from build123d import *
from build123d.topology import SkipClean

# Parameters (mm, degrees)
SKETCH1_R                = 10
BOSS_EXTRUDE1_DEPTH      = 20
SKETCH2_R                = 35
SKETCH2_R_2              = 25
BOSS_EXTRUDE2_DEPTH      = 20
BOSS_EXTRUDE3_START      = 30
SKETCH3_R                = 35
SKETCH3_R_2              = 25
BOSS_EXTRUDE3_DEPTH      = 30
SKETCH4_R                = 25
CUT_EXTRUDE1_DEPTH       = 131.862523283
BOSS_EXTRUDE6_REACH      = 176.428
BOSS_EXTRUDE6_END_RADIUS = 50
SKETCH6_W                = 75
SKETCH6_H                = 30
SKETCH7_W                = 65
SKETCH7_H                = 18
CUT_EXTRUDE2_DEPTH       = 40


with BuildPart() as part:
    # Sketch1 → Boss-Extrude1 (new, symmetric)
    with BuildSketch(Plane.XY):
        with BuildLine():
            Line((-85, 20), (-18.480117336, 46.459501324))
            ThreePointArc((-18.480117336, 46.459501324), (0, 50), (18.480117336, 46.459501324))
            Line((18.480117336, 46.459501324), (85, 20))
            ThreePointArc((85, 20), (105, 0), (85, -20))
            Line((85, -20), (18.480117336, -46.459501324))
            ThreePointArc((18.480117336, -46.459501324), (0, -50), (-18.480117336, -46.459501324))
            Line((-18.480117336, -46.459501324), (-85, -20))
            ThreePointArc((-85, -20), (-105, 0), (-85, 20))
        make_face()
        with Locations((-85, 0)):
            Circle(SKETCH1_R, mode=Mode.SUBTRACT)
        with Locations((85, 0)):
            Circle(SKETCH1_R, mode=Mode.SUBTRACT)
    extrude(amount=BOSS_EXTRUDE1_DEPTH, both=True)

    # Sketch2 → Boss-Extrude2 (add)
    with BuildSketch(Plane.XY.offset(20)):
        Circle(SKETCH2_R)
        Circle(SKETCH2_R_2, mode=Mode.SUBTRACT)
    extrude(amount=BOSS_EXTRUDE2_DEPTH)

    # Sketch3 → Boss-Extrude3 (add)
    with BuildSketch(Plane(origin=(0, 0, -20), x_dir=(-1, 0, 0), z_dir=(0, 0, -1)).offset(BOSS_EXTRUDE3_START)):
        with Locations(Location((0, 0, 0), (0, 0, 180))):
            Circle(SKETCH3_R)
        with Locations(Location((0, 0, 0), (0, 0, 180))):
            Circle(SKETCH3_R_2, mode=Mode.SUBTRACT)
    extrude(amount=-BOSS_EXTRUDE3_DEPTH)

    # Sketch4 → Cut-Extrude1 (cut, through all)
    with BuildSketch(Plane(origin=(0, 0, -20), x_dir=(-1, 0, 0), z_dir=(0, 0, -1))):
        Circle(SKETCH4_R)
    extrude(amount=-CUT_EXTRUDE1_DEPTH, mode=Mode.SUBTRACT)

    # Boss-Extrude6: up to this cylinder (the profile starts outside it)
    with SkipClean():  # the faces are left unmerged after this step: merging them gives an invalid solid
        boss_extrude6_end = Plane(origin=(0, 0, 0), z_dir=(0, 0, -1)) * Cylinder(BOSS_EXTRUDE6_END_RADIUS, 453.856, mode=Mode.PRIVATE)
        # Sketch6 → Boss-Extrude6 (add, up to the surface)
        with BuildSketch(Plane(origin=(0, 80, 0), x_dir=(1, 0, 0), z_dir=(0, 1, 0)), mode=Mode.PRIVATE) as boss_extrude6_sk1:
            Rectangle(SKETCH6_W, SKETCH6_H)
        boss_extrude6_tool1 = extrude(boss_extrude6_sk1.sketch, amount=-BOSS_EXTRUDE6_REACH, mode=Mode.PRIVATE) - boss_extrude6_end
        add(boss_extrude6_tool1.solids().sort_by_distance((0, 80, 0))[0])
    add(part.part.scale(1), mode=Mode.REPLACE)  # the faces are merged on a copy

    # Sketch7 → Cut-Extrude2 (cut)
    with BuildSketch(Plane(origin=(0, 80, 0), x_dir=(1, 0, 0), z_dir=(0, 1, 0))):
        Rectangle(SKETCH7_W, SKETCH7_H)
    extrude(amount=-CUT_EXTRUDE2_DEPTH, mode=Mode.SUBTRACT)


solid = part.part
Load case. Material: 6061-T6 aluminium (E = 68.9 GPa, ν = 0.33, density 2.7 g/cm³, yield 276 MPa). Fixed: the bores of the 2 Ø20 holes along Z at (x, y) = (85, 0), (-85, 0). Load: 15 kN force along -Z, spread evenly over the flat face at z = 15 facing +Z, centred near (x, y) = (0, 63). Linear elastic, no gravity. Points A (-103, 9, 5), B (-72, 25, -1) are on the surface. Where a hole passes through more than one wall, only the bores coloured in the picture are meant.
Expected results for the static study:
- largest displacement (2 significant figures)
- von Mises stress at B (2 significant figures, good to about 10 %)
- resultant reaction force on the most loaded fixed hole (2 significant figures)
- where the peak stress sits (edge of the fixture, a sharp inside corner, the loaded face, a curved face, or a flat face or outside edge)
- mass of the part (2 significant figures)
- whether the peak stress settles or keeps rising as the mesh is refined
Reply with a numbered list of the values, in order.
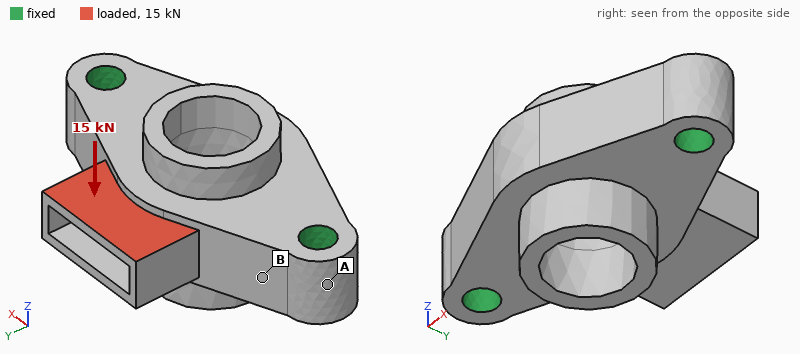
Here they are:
1. 0.48 mm
2. 38 MPa
3. 7.5 kN
4. a sharp inside corner
5. 1.5 kg
6. keeps rising
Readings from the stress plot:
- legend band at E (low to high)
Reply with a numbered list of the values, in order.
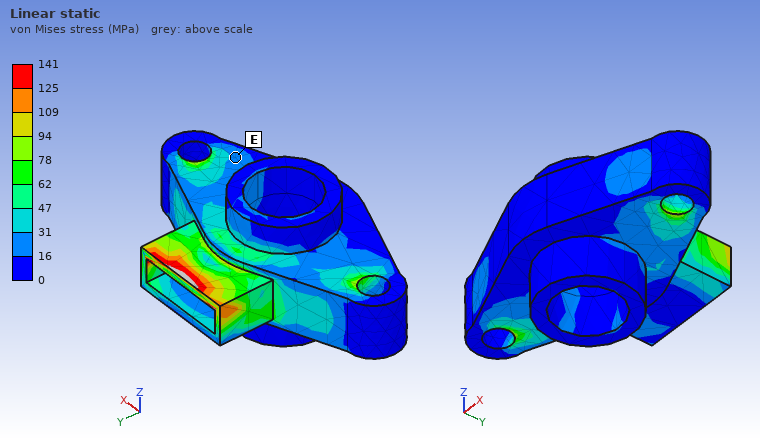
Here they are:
1. 16 to 31 MPa
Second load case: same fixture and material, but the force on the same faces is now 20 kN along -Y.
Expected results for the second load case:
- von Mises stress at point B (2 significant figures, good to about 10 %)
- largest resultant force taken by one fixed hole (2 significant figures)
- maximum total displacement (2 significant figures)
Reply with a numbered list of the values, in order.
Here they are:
1. 10 MPa
2. 11 kN
3. 0.15 mm
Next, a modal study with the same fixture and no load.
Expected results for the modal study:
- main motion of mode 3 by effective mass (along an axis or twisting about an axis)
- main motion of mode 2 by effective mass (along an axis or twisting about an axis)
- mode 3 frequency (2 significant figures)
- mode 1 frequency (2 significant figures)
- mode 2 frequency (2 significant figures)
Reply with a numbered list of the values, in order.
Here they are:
1. along Y
2. along Z
3. 5700 Hz
4. 3400 Hz
5. 4500 Hz
